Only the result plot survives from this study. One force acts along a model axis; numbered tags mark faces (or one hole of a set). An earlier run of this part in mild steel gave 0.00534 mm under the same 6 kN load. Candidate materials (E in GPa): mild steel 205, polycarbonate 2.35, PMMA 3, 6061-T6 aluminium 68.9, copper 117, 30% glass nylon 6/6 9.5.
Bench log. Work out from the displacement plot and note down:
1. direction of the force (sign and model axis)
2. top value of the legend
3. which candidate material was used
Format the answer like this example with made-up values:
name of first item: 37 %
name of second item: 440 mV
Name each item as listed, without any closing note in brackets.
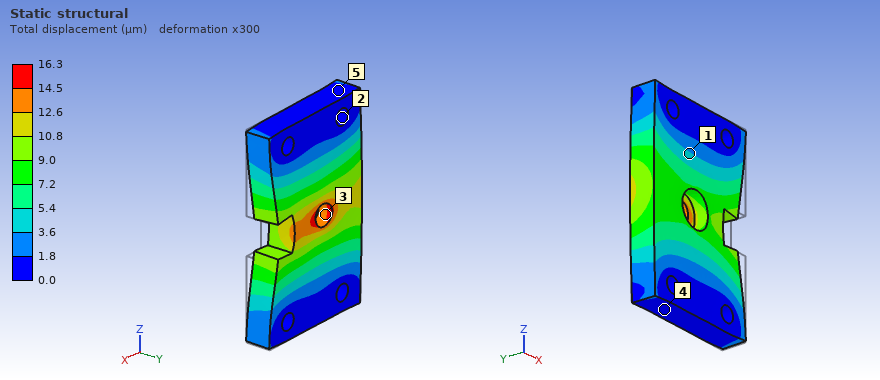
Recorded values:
direction of the force: -X
top value of the legend: 16.3 µm
which candidate material was used: 6061-T6 aluminium
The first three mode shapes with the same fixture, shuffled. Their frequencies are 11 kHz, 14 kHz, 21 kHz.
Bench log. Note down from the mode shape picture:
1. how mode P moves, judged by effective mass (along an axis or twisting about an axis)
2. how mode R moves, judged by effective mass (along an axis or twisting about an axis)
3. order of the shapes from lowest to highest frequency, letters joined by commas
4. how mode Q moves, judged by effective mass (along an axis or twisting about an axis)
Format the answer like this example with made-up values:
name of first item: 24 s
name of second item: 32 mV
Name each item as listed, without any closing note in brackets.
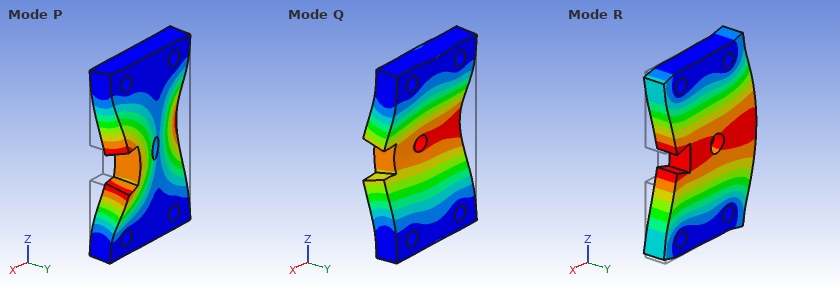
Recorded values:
how mode P moves, judged by effective mass: twisting about Z
how mode R moves, judged by effective mass: along X
order of the shapes from lowest to highest frequency, letters joined by commas: Q, P, R
how mode Q moves, judged by effective mass: along Y
